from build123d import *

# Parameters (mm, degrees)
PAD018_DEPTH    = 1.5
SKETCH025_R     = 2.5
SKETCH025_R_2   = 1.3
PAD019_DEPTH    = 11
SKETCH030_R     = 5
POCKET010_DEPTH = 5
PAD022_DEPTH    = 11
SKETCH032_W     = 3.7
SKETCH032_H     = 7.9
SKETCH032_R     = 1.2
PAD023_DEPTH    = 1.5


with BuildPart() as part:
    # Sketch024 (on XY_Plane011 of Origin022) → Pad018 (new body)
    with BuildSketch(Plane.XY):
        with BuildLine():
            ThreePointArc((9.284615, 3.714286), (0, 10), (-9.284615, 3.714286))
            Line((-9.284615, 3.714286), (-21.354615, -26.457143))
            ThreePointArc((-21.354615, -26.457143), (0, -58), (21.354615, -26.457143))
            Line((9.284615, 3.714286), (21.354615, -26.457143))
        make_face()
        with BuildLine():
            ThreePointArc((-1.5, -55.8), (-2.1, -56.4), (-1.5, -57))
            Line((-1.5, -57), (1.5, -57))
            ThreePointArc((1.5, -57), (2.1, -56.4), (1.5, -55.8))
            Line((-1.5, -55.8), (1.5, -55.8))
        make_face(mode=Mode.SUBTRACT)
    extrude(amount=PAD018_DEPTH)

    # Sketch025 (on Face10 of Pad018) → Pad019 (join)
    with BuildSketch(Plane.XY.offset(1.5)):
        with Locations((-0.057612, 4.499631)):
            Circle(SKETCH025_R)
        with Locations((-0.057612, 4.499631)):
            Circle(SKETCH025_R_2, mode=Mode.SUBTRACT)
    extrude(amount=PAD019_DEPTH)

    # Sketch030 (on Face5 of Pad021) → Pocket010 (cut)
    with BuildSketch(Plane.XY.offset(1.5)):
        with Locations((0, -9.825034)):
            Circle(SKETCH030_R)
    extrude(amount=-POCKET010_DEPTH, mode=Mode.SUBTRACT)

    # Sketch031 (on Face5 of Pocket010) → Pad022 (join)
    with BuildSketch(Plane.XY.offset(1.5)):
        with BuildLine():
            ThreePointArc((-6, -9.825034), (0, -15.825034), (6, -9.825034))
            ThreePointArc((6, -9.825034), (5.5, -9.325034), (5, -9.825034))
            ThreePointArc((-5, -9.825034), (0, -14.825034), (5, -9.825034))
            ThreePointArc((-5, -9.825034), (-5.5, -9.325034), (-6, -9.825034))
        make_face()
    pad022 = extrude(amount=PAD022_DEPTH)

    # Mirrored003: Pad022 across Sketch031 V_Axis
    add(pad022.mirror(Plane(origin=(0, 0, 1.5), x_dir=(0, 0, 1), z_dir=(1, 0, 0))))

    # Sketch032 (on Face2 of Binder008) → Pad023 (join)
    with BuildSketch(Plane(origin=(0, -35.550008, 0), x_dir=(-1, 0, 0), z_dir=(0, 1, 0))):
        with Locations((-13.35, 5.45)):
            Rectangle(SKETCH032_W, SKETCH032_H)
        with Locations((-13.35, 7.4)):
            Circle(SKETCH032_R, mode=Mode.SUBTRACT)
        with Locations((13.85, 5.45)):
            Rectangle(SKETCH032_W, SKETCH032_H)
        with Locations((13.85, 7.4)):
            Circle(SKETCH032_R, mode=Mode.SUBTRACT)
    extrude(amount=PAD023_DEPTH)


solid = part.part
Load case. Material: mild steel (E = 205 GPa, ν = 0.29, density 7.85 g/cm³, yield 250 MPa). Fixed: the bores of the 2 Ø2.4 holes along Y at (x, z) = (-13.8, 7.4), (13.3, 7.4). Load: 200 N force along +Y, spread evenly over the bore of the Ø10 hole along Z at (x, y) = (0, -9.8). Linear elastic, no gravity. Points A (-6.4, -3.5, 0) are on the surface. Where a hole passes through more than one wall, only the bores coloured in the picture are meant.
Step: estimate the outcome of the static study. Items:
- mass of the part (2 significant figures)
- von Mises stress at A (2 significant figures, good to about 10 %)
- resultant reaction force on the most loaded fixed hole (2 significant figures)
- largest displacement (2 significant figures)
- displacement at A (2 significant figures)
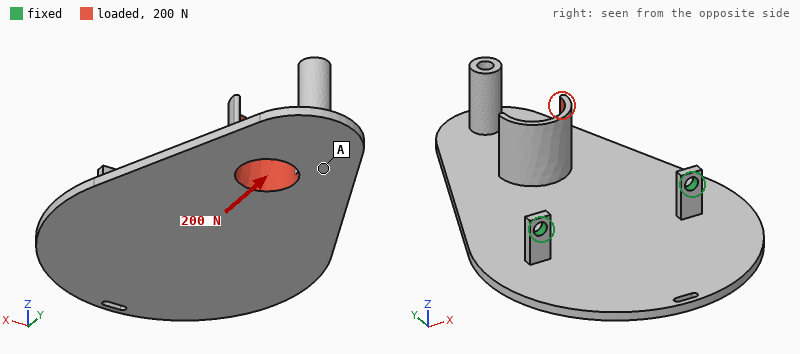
29 g
17 MPa
100 N
0.52 mm
0.33 mm
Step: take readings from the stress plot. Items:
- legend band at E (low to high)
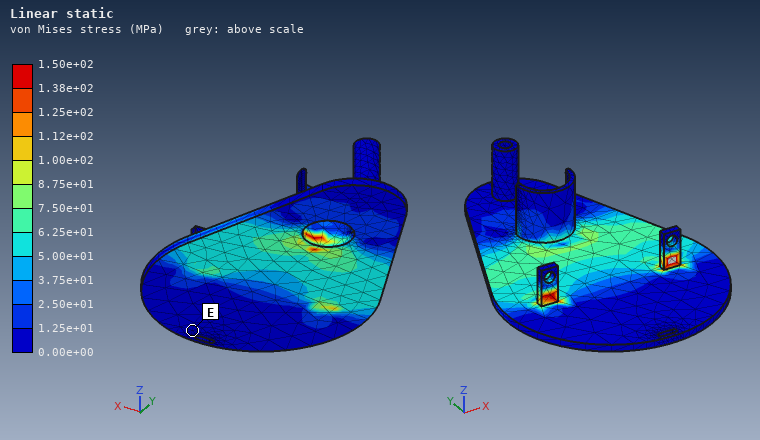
0.00e+00 to 1.25e+01 MPa
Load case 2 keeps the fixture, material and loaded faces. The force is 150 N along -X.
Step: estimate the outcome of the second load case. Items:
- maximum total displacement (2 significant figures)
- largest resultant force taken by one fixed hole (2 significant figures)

0.12 mm
140 N
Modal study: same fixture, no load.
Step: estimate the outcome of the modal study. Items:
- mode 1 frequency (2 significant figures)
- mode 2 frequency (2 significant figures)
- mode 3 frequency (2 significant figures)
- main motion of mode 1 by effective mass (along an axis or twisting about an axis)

380 Hz
1700 Hz
2000 Hz
along Z
